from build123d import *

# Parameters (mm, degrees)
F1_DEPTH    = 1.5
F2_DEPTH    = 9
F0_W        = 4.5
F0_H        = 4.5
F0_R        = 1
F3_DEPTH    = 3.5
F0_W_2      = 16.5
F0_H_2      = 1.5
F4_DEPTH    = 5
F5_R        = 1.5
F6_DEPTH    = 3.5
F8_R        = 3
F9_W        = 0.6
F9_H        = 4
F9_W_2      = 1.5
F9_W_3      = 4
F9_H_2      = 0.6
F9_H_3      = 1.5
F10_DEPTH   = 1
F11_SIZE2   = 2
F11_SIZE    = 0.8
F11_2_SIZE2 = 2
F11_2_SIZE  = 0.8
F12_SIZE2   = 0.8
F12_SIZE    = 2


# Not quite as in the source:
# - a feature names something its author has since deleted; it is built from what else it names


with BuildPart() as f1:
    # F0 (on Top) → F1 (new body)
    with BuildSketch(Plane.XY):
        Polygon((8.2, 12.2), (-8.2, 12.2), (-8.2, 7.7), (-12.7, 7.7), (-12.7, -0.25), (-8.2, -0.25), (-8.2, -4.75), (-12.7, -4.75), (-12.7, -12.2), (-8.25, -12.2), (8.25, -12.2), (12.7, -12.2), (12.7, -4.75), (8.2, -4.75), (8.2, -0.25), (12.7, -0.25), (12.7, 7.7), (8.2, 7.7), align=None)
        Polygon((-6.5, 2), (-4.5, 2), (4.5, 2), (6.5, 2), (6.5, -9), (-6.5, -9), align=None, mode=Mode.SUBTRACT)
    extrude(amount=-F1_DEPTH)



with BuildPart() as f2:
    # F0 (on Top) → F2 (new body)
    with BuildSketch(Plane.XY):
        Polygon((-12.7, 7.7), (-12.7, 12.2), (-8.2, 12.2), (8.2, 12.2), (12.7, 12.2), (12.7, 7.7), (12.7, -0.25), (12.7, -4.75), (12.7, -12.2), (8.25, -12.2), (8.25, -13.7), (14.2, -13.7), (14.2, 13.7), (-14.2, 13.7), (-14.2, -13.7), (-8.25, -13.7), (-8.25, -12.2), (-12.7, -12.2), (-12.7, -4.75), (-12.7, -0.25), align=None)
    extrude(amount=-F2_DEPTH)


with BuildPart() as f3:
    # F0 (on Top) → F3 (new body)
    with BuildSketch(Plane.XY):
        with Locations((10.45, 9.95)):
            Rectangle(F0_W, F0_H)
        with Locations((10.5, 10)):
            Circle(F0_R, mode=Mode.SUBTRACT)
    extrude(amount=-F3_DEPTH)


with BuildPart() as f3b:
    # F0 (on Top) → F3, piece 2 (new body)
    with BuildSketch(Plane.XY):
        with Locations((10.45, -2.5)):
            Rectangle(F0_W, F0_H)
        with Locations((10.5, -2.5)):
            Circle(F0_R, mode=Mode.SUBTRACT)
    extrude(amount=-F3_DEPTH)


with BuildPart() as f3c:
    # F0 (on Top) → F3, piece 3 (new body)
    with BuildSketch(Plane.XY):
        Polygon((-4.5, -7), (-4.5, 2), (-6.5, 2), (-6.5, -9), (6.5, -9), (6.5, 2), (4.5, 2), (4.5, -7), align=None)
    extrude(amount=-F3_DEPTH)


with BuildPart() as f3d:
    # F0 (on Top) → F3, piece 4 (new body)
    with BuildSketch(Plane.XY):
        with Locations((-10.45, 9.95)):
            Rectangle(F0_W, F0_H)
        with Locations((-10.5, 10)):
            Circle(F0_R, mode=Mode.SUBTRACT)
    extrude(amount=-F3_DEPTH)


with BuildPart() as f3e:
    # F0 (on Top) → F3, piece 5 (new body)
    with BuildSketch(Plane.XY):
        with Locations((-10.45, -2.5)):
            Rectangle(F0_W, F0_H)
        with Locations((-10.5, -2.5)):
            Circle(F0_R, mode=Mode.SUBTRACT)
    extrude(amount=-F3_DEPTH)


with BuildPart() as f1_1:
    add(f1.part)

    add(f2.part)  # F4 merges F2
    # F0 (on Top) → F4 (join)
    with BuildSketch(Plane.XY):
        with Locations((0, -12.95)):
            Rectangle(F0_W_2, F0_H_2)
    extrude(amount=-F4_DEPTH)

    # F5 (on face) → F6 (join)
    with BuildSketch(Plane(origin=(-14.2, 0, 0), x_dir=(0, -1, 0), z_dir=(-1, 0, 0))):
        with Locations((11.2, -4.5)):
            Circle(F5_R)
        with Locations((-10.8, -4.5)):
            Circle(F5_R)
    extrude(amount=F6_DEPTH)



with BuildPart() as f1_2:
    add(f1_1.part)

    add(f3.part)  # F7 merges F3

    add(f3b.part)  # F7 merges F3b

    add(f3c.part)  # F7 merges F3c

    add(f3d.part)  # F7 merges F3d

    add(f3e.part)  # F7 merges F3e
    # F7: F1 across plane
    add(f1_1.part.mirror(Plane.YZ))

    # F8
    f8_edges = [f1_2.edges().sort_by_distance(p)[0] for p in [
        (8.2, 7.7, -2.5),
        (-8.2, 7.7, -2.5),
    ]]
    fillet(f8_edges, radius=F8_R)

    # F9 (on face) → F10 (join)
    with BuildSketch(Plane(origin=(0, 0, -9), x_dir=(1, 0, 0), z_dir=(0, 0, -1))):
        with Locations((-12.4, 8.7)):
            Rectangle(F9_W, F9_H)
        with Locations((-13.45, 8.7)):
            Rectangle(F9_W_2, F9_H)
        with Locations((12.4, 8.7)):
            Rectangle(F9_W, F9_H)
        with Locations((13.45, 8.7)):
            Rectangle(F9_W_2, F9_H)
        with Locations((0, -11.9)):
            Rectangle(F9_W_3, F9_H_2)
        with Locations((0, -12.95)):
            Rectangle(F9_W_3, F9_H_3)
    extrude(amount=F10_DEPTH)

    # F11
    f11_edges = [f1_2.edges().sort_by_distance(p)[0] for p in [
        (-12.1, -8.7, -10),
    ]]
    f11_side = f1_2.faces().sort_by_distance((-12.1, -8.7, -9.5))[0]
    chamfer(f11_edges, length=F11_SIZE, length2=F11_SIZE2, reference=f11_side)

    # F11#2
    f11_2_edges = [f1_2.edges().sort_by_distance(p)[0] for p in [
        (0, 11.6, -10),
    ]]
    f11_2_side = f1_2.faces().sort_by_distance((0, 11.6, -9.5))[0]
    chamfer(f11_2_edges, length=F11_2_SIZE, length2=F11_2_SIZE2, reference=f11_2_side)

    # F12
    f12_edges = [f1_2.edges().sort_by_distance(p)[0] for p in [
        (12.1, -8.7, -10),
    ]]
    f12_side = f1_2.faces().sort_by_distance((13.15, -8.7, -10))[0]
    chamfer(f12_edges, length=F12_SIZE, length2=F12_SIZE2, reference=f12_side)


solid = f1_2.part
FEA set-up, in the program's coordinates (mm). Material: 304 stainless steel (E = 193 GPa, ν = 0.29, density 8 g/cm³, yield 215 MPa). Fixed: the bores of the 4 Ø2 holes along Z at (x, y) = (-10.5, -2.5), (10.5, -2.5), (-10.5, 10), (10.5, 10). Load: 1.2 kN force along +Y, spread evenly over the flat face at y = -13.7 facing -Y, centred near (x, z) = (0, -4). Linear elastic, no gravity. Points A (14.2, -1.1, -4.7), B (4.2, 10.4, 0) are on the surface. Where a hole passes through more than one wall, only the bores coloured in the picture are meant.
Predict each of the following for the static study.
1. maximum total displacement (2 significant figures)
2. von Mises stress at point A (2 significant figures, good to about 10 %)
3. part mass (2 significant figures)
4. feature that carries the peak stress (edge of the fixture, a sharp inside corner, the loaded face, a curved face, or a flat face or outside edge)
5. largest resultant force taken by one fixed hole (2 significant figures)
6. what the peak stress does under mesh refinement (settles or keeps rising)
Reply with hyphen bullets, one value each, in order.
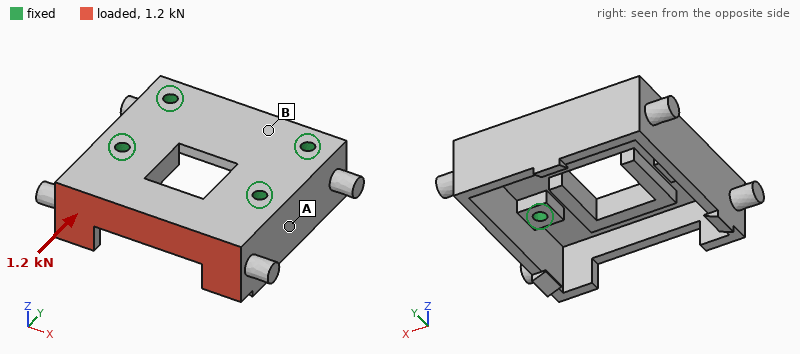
- 21 µm
- 35 MPa
- 20 g
- a sharp inside corner
- 450 N
- keeps rising
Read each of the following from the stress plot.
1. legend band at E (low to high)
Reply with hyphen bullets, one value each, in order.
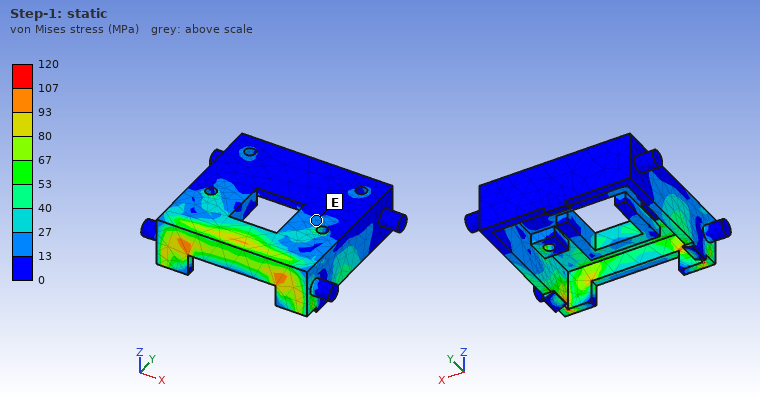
- 13 to 27 MPa
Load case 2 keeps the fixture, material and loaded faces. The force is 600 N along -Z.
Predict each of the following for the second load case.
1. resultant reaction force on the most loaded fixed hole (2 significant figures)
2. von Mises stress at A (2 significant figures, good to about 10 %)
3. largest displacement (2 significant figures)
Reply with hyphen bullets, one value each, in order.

- 490 N
- 44 MPa
- 31 µm
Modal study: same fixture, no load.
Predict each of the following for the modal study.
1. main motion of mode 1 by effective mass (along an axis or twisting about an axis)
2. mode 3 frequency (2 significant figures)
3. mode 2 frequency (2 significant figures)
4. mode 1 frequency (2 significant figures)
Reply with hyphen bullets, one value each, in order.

- along Z
- 19 kHz
- 18 kHz
- 14 kHz
